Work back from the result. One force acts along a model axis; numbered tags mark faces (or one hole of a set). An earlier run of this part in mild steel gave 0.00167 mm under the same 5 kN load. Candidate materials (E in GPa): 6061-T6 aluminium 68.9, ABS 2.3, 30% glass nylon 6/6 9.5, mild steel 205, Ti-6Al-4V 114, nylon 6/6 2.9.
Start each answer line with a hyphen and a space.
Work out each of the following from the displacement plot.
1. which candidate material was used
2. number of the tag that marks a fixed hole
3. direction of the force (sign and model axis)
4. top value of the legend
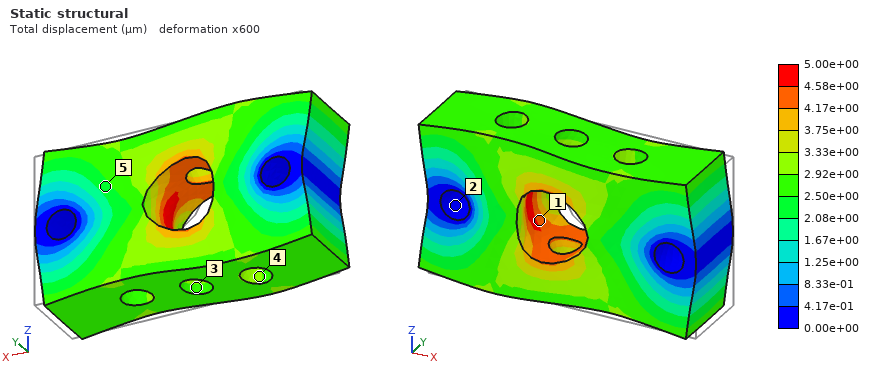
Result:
- 6061-T6 aluminium
- 2
- -X
- 5.00e+00 µm
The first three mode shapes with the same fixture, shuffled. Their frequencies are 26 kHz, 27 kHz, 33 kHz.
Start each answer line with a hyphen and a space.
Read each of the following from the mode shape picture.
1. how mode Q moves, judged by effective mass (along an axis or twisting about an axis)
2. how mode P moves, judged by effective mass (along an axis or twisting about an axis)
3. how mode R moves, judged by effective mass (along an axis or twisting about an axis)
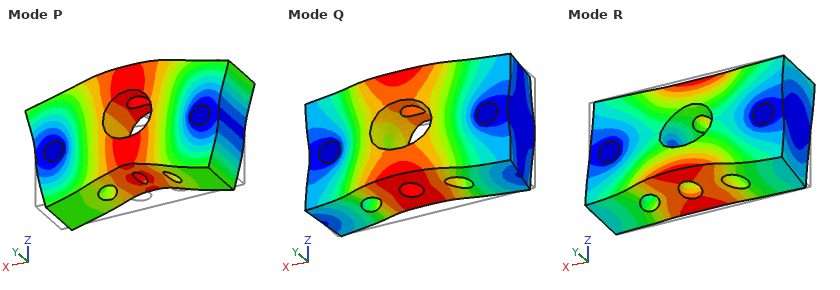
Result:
- along Y
- along Z
- twisting about X
